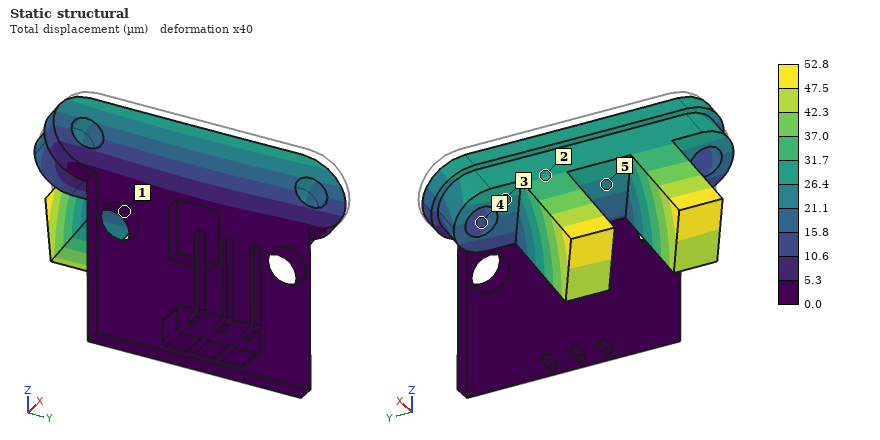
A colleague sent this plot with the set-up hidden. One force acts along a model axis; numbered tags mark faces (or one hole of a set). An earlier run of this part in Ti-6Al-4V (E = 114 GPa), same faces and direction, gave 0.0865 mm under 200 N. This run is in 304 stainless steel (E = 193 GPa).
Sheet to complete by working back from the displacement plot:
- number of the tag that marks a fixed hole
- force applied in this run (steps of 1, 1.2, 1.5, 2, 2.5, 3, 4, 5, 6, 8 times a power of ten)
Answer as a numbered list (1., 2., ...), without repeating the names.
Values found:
1. 1
2. 200 N
